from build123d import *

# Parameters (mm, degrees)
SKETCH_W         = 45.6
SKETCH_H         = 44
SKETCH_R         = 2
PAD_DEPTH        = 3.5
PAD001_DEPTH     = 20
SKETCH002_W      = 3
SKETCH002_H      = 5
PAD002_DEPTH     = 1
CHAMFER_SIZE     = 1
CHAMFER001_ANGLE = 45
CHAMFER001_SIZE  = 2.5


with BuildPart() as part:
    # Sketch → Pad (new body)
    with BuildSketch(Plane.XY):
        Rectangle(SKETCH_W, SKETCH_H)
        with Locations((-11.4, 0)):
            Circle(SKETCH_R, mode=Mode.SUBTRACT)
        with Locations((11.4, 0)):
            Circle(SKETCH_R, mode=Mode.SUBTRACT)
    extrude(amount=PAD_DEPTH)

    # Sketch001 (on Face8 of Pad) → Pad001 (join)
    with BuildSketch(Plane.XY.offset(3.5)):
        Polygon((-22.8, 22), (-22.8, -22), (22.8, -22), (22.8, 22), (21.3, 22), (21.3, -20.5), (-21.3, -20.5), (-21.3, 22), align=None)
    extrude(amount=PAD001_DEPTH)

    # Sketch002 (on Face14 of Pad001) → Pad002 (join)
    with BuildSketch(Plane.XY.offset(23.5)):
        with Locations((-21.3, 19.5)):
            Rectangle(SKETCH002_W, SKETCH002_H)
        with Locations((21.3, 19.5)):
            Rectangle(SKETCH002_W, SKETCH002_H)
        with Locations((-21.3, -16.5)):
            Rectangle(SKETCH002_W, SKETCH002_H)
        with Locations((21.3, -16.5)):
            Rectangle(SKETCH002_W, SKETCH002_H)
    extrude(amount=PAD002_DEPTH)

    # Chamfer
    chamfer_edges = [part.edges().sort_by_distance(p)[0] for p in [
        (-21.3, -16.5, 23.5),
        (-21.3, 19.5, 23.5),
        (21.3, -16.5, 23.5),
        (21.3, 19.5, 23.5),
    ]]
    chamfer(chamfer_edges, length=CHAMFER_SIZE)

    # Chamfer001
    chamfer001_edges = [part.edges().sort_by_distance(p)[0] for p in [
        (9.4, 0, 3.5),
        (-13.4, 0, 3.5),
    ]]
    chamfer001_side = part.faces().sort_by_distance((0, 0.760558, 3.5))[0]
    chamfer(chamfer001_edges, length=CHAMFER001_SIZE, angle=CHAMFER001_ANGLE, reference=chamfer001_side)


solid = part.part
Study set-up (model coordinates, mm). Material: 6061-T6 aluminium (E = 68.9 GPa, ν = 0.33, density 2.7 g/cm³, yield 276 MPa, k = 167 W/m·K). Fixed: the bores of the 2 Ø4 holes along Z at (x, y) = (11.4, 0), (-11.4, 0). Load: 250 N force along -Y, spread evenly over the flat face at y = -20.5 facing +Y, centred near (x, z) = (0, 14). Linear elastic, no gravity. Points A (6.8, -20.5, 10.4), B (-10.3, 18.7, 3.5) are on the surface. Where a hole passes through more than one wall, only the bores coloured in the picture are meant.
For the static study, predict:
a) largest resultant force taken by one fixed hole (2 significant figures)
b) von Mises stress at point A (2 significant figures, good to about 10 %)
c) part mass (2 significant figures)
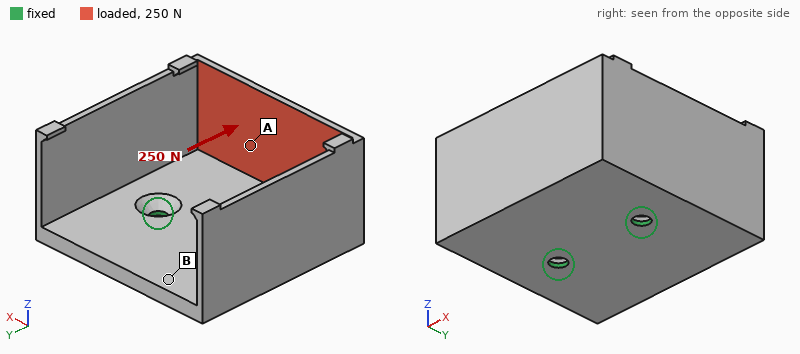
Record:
130 N
21 MPa
29 g
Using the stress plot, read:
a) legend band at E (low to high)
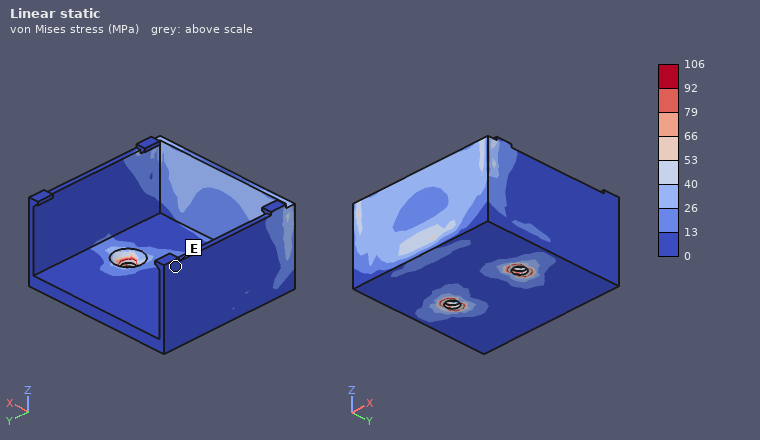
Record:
0 to 13 MPa
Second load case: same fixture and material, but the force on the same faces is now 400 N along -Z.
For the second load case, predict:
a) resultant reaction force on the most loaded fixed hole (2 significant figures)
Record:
220 N
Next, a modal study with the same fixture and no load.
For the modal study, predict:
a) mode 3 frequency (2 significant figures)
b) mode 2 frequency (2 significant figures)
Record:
3000 Hz
2800 Hz
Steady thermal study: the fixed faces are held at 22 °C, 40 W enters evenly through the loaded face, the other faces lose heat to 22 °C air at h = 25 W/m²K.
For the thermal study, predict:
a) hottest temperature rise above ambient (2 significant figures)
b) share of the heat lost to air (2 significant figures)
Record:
58 K
12 %
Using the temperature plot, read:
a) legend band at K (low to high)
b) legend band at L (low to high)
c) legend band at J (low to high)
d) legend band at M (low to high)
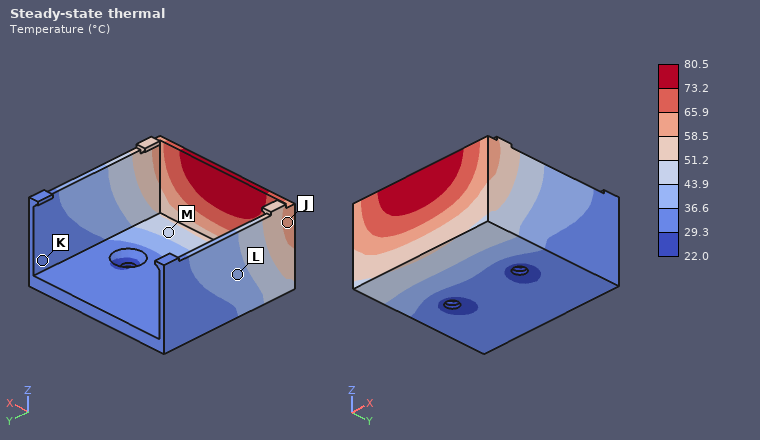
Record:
29.3 to 36.6 °C
36.6 to 43.9 °C
58.5 to 65.9 °C
43.9 to 51.2 °C
